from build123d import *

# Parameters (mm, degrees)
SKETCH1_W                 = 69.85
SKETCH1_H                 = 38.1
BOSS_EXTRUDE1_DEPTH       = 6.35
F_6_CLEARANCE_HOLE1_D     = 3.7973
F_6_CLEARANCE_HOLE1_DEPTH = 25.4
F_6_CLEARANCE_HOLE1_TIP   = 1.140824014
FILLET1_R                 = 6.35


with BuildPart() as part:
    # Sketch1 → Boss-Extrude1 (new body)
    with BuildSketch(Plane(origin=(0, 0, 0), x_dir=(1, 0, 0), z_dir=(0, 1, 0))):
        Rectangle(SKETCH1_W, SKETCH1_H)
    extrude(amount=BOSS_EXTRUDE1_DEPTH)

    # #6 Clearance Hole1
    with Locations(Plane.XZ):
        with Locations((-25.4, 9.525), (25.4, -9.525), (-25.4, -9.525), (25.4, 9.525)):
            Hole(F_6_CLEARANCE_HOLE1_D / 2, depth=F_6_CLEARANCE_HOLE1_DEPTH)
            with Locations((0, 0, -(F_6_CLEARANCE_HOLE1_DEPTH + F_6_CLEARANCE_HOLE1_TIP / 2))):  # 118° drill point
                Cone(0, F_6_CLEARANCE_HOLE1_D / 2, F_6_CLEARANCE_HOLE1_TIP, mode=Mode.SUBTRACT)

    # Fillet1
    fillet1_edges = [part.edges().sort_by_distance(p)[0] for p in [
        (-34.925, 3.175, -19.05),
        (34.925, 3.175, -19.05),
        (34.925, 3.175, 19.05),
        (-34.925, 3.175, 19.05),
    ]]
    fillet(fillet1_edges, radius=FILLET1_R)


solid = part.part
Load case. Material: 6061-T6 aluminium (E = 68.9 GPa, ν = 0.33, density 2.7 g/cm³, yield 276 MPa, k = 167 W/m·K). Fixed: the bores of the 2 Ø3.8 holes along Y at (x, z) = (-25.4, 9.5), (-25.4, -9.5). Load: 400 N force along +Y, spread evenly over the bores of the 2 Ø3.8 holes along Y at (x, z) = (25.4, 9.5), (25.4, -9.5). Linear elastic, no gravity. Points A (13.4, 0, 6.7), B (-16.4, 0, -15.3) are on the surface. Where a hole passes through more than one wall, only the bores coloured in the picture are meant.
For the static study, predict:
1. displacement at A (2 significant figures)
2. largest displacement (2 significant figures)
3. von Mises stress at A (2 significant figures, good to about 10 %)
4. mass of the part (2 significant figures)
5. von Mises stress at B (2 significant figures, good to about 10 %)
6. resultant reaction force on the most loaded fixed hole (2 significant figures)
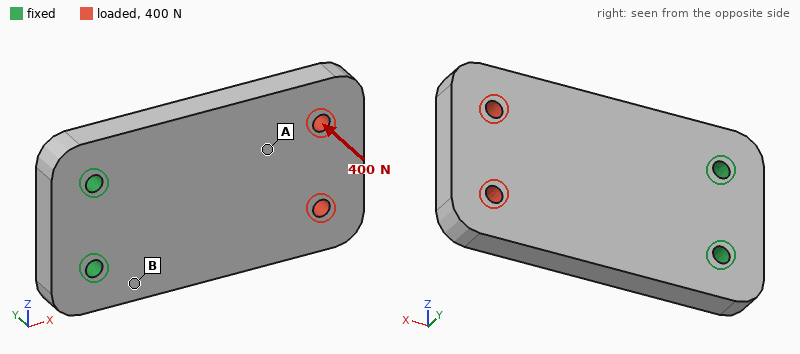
0.21 mm
0.41 mm
19 MPa
44 g
61 MPa
200 N
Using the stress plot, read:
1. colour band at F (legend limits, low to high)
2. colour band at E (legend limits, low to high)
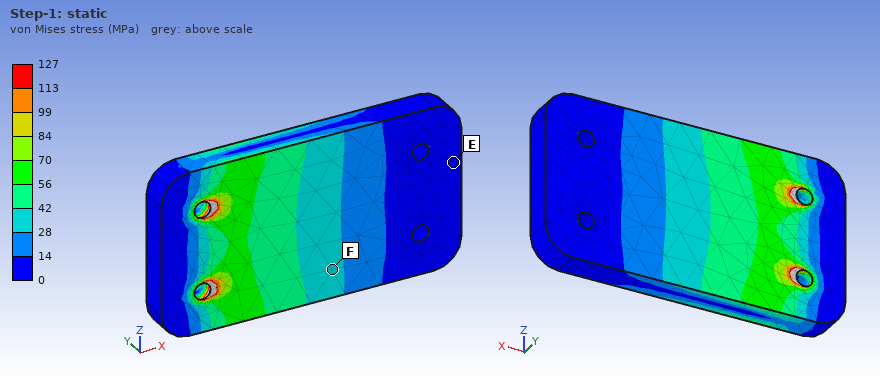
28 to 42 MPa
0 to 14 MPa
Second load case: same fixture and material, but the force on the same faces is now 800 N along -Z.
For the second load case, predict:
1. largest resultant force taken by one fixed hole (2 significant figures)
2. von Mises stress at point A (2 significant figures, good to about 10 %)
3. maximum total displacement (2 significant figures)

1.9 kN
7.9 MPa
41 µm
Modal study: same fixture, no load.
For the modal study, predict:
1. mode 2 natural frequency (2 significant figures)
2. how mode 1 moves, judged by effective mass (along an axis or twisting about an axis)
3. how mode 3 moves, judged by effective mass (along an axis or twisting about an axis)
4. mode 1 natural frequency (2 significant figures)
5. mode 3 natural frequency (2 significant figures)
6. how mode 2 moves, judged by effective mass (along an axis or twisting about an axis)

4700 Hz
along Y
along Z
1400 Hz
5900 Hz
twisting about X
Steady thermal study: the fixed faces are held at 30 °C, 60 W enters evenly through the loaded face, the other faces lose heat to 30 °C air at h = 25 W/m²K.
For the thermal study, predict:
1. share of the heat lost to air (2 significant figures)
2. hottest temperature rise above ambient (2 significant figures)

9.8 %
77 K
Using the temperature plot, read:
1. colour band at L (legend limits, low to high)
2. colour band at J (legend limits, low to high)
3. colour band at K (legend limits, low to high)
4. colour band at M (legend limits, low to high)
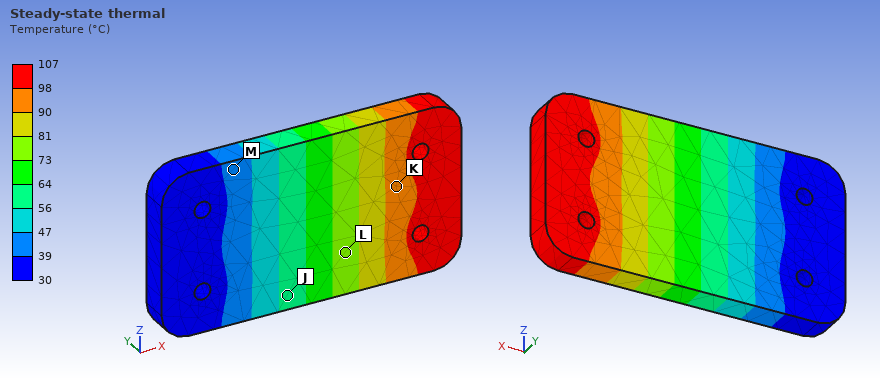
73 to 81 °C
56 to 64 °C
90 to 98 °C
39 to 47 °C
